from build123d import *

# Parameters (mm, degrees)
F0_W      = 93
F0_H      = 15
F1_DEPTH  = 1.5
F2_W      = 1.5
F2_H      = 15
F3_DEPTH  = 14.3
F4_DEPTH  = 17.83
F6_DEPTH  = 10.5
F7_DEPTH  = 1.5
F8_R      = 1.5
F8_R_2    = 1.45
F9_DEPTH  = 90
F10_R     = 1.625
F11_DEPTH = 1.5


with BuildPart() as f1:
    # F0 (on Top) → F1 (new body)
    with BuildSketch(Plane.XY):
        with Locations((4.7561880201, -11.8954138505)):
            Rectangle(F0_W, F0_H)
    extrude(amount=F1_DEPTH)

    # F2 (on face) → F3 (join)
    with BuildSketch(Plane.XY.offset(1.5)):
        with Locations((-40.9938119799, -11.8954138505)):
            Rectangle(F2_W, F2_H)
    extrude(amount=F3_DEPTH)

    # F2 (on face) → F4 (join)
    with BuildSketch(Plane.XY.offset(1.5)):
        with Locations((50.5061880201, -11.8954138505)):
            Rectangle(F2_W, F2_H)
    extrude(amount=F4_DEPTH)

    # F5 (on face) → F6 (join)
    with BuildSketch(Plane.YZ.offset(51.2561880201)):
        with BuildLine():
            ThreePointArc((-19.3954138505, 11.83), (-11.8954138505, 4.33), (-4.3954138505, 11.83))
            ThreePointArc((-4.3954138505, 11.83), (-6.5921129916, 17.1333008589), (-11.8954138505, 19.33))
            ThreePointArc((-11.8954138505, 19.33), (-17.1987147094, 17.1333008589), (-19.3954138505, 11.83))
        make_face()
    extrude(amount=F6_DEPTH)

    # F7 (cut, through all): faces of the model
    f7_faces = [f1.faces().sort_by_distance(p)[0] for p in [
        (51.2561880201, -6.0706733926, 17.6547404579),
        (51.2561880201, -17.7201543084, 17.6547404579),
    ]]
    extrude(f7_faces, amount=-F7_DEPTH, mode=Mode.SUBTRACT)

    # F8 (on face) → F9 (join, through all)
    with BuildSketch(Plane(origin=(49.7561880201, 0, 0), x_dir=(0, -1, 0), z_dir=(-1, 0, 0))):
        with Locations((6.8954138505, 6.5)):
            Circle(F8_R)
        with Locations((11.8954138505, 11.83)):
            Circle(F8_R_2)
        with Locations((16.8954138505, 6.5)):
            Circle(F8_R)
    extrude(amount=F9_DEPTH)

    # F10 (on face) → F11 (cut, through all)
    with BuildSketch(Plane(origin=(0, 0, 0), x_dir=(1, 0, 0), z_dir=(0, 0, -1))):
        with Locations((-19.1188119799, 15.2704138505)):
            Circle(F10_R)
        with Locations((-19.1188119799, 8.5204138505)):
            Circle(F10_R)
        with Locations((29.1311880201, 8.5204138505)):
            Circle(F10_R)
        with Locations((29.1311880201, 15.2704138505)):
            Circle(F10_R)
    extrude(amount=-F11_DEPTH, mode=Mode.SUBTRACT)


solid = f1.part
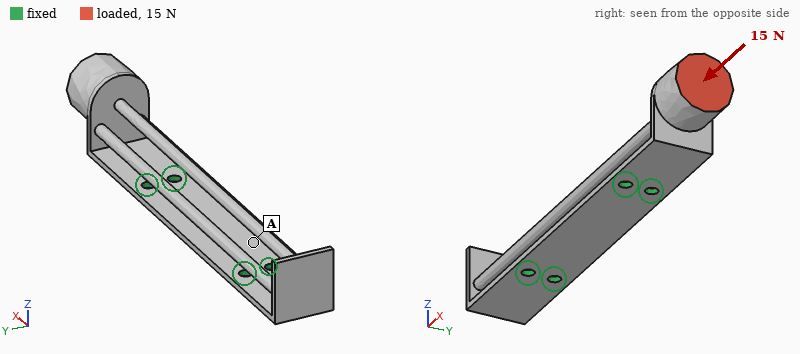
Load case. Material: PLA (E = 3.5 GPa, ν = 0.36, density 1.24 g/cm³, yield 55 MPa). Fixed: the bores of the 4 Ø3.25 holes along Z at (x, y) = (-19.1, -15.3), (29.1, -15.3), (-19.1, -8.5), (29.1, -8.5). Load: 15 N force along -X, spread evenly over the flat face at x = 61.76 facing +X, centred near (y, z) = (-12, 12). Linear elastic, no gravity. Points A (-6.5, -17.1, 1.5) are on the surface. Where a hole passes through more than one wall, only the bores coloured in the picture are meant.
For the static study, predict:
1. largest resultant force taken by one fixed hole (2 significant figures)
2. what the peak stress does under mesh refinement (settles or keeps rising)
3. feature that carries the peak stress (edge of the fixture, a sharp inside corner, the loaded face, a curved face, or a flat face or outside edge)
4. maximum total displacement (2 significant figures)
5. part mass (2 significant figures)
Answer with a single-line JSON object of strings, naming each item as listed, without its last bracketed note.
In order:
{"largest resultant force taken by one fixed hole": "4.5 N", "what the peak stress does under mesh refinement": "keeps rising", "feature that carries the peak stress": "edge of the fixture", "maximum total displacement": "1.1 mm", "part mass": "8.0 g"}
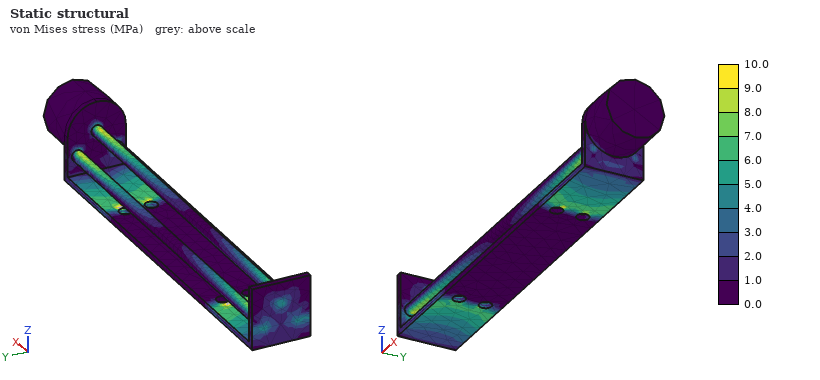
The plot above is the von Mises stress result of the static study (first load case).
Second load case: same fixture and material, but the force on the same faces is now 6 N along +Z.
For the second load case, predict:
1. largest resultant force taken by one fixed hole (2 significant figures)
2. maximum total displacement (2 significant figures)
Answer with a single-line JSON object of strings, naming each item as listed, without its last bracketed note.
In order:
{"largest resultant force taken by one fixed hole": "5.1 N", "maximum total displacement": "1.2 mm"}
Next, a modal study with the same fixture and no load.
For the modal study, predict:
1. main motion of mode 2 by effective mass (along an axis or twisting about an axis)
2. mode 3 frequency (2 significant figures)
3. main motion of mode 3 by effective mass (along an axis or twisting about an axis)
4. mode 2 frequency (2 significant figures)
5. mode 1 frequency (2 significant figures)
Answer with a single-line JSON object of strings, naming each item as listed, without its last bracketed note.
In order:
{"main motion of mode 2 by effective mass": "along Y", "mode 3 frequency": "370 Hz", "main motion of mode 3 by effective mass": "along Z", "mode 2 frequency": "280 Hz", "mode 1 frequency": "240 Hz"}
